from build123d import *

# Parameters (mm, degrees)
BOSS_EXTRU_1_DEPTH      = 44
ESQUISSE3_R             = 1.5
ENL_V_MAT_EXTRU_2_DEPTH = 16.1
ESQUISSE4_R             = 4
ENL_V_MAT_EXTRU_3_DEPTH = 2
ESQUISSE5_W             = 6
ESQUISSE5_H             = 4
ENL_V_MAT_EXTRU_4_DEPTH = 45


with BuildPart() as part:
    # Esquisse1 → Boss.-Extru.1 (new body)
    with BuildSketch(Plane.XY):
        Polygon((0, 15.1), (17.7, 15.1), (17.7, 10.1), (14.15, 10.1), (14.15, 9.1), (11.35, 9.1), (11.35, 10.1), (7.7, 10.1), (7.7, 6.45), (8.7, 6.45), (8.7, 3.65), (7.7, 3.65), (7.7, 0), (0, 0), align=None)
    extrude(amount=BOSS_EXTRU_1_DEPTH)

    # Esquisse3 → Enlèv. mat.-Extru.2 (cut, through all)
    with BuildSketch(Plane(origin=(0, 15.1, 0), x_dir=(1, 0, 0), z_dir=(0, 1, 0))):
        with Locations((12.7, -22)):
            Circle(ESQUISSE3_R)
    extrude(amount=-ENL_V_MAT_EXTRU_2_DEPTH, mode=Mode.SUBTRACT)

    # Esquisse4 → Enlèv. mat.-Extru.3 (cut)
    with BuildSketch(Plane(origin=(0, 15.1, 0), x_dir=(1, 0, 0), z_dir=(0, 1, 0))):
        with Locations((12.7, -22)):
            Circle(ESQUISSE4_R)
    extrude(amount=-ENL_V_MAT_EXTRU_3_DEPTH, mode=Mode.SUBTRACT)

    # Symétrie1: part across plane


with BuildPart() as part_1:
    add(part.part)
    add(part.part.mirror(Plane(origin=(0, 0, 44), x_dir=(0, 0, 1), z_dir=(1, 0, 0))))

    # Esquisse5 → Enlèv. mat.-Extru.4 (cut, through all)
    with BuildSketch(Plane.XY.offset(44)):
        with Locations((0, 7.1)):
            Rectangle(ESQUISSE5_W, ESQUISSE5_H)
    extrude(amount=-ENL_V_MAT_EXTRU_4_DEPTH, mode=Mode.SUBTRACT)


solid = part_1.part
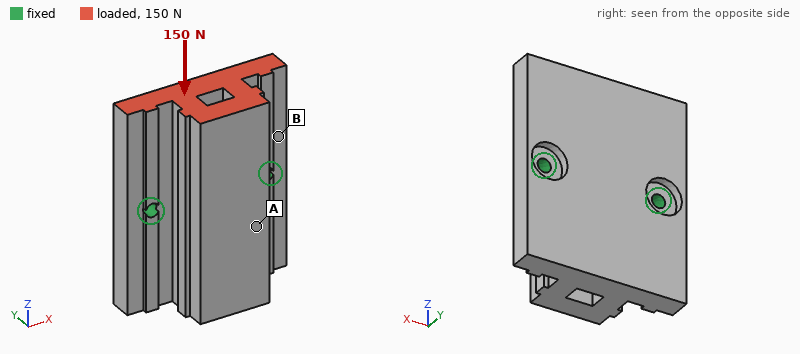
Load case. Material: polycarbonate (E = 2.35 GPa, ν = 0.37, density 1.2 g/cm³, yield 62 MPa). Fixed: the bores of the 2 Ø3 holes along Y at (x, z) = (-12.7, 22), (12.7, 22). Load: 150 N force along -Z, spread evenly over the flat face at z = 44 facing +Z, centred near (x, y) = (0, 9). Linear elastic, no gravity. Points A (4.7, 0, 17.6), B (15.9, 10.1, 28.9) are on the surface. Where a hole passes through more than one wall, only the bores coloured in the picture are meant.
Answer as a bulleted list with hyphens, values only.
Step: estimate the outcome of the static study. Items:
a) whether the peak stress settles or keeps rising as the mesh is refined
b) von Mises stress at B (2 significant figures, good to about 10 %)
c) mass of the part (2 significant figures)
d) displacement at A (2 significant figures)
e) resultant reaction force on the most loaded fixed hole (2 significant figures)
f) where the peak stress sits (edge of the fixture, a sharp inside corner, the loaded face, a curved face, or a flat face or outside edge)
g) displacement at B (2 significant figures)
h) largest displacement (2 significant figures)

- keeps rising
- 1.4 MPa
- 17 g
- 39 µm
- 75 N
- edge of the fixture
- 14 µm
- 74 µm
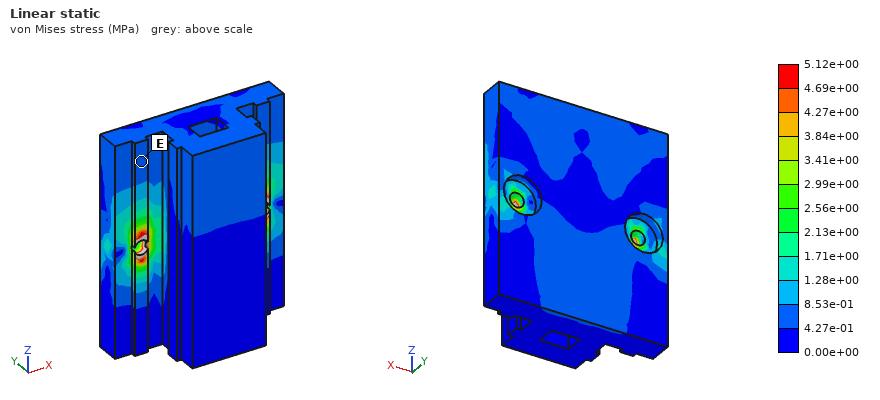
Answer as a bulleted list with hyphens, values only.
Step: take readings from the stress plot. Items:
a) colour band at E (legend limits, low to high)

- 4.27e-01 to 8.53e-01 MPa
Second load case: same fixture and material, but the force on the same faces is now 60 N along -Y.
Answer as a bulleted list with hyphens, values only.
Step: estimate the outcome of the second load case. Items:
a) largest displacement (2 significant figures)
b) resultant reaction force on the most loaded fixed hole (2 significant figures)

- 0.29 mm
- 31 N
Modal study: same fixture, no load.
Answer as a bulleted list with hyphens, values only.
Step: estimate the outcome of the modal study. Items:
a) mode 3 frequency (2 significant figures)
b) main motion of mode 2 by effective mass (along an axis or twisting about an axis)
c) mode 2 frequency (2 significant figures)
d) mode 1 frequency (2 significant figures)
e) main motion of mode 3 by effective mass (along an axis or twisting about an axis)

- 3800 Hz
- along Y
- 3000 Hz
- 1000 Hz
- along X
